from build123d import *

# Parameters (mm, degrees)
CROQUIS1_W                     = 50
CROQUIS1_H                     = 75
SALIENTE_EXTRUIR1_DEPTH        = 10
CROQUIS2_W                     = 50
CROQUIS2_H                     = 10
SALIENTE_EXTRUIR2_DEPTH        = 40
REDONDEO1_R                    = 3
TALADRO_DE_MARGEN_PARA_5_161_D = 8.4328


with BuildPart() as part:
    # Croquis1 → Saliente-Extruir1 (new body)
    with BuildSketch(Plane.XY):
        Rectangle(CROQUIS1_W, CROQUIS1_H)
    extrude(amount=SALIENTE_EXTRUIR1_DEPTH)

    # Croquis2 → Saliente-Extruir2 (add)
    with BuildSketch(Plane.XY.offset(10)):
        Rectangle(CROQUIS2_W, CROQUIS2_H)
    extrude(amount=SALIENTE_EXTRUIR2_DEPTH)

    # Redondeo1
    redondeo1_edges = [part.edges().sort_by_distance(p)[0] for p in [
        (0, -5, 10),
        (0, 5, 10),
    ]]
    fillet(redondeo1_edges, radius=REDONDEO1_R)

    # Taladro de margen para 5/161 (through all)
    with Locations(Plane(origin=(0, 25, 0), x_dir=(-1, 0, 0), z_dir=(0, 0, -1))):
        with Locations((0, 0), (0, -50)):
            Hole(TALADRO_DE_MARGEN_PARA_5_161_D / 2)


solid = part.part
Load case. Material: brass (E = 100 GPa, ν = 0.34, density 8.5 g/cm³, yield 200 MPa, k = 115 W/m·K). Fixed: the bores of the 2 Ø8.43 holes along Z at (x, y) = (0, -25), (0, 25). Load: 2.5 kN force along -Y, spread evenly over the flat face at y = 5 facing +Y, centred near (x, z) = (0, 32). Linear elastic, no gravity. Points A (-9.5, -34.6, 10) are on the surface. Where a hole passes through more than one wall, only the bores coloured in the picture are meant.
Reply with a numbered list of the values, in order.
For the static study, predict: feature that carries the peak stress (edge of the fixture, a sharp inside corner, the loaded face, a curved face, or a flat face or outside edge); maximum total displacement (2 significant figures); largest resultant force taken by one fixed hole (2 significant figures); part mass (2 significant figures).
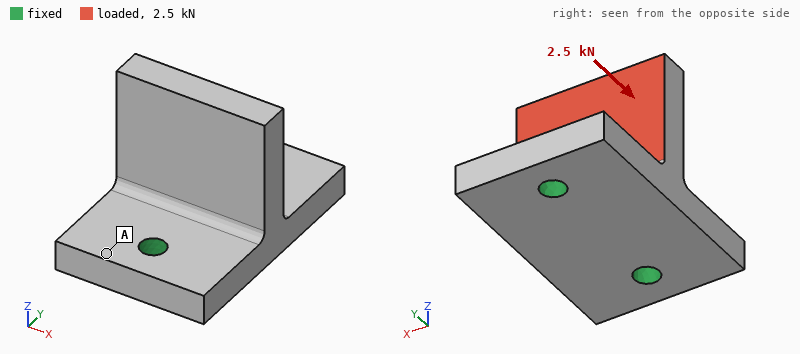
1. a curved face
2. 78 µm
3. 2.1 kN
4. 480 g
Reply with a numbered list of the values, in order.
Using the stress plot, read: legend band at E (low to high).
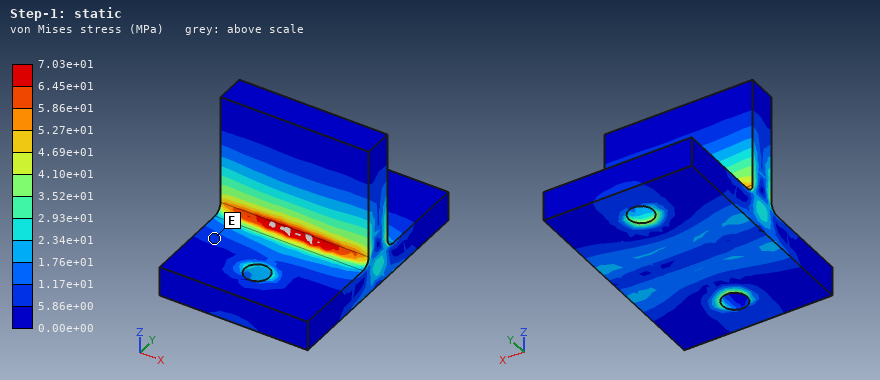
1. 5.86e+00 to 1.17e+01 MPa
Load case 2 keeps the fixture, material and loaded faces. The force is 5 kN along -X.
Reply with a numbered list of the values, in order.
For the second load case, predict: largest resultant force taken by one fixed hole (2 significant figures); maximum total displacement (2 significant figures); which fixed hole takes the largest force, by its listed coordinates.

1. 3.0 kN
2. 0.12 mm
3. (0, 25)
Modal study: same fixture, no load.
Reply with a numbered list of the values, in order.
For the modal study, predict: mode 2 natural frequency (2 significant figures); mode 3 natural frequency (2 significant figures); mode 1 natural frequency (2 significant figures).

1. 2800 Hz
2. 5600 Hz
3. 2800 Hz
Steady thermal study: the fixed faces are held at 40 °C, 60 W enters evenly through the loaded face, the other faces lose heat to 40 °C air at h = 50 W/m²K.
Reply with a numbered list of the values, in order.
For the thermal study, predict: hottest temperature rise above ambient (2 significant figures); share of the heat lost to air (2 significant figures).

1. 35 K
2. 12 %
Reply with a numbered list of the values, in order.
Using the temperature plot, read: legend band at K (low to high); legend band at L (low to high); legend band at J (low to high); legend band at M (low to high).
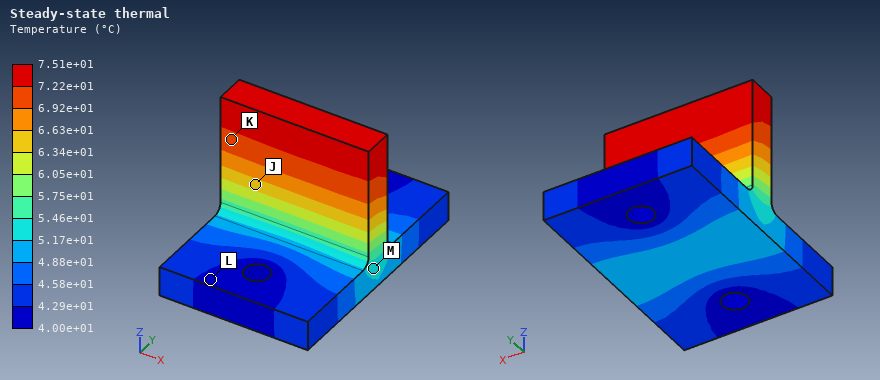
1. 6.92e+01 to 7.22e+01 °C
2. 4.00e+01 to 4.29e+01 °C
3. 6.34e+01 to 6.63e+01 °C
4. 5.17e+01 to 5.46e+01 °C
